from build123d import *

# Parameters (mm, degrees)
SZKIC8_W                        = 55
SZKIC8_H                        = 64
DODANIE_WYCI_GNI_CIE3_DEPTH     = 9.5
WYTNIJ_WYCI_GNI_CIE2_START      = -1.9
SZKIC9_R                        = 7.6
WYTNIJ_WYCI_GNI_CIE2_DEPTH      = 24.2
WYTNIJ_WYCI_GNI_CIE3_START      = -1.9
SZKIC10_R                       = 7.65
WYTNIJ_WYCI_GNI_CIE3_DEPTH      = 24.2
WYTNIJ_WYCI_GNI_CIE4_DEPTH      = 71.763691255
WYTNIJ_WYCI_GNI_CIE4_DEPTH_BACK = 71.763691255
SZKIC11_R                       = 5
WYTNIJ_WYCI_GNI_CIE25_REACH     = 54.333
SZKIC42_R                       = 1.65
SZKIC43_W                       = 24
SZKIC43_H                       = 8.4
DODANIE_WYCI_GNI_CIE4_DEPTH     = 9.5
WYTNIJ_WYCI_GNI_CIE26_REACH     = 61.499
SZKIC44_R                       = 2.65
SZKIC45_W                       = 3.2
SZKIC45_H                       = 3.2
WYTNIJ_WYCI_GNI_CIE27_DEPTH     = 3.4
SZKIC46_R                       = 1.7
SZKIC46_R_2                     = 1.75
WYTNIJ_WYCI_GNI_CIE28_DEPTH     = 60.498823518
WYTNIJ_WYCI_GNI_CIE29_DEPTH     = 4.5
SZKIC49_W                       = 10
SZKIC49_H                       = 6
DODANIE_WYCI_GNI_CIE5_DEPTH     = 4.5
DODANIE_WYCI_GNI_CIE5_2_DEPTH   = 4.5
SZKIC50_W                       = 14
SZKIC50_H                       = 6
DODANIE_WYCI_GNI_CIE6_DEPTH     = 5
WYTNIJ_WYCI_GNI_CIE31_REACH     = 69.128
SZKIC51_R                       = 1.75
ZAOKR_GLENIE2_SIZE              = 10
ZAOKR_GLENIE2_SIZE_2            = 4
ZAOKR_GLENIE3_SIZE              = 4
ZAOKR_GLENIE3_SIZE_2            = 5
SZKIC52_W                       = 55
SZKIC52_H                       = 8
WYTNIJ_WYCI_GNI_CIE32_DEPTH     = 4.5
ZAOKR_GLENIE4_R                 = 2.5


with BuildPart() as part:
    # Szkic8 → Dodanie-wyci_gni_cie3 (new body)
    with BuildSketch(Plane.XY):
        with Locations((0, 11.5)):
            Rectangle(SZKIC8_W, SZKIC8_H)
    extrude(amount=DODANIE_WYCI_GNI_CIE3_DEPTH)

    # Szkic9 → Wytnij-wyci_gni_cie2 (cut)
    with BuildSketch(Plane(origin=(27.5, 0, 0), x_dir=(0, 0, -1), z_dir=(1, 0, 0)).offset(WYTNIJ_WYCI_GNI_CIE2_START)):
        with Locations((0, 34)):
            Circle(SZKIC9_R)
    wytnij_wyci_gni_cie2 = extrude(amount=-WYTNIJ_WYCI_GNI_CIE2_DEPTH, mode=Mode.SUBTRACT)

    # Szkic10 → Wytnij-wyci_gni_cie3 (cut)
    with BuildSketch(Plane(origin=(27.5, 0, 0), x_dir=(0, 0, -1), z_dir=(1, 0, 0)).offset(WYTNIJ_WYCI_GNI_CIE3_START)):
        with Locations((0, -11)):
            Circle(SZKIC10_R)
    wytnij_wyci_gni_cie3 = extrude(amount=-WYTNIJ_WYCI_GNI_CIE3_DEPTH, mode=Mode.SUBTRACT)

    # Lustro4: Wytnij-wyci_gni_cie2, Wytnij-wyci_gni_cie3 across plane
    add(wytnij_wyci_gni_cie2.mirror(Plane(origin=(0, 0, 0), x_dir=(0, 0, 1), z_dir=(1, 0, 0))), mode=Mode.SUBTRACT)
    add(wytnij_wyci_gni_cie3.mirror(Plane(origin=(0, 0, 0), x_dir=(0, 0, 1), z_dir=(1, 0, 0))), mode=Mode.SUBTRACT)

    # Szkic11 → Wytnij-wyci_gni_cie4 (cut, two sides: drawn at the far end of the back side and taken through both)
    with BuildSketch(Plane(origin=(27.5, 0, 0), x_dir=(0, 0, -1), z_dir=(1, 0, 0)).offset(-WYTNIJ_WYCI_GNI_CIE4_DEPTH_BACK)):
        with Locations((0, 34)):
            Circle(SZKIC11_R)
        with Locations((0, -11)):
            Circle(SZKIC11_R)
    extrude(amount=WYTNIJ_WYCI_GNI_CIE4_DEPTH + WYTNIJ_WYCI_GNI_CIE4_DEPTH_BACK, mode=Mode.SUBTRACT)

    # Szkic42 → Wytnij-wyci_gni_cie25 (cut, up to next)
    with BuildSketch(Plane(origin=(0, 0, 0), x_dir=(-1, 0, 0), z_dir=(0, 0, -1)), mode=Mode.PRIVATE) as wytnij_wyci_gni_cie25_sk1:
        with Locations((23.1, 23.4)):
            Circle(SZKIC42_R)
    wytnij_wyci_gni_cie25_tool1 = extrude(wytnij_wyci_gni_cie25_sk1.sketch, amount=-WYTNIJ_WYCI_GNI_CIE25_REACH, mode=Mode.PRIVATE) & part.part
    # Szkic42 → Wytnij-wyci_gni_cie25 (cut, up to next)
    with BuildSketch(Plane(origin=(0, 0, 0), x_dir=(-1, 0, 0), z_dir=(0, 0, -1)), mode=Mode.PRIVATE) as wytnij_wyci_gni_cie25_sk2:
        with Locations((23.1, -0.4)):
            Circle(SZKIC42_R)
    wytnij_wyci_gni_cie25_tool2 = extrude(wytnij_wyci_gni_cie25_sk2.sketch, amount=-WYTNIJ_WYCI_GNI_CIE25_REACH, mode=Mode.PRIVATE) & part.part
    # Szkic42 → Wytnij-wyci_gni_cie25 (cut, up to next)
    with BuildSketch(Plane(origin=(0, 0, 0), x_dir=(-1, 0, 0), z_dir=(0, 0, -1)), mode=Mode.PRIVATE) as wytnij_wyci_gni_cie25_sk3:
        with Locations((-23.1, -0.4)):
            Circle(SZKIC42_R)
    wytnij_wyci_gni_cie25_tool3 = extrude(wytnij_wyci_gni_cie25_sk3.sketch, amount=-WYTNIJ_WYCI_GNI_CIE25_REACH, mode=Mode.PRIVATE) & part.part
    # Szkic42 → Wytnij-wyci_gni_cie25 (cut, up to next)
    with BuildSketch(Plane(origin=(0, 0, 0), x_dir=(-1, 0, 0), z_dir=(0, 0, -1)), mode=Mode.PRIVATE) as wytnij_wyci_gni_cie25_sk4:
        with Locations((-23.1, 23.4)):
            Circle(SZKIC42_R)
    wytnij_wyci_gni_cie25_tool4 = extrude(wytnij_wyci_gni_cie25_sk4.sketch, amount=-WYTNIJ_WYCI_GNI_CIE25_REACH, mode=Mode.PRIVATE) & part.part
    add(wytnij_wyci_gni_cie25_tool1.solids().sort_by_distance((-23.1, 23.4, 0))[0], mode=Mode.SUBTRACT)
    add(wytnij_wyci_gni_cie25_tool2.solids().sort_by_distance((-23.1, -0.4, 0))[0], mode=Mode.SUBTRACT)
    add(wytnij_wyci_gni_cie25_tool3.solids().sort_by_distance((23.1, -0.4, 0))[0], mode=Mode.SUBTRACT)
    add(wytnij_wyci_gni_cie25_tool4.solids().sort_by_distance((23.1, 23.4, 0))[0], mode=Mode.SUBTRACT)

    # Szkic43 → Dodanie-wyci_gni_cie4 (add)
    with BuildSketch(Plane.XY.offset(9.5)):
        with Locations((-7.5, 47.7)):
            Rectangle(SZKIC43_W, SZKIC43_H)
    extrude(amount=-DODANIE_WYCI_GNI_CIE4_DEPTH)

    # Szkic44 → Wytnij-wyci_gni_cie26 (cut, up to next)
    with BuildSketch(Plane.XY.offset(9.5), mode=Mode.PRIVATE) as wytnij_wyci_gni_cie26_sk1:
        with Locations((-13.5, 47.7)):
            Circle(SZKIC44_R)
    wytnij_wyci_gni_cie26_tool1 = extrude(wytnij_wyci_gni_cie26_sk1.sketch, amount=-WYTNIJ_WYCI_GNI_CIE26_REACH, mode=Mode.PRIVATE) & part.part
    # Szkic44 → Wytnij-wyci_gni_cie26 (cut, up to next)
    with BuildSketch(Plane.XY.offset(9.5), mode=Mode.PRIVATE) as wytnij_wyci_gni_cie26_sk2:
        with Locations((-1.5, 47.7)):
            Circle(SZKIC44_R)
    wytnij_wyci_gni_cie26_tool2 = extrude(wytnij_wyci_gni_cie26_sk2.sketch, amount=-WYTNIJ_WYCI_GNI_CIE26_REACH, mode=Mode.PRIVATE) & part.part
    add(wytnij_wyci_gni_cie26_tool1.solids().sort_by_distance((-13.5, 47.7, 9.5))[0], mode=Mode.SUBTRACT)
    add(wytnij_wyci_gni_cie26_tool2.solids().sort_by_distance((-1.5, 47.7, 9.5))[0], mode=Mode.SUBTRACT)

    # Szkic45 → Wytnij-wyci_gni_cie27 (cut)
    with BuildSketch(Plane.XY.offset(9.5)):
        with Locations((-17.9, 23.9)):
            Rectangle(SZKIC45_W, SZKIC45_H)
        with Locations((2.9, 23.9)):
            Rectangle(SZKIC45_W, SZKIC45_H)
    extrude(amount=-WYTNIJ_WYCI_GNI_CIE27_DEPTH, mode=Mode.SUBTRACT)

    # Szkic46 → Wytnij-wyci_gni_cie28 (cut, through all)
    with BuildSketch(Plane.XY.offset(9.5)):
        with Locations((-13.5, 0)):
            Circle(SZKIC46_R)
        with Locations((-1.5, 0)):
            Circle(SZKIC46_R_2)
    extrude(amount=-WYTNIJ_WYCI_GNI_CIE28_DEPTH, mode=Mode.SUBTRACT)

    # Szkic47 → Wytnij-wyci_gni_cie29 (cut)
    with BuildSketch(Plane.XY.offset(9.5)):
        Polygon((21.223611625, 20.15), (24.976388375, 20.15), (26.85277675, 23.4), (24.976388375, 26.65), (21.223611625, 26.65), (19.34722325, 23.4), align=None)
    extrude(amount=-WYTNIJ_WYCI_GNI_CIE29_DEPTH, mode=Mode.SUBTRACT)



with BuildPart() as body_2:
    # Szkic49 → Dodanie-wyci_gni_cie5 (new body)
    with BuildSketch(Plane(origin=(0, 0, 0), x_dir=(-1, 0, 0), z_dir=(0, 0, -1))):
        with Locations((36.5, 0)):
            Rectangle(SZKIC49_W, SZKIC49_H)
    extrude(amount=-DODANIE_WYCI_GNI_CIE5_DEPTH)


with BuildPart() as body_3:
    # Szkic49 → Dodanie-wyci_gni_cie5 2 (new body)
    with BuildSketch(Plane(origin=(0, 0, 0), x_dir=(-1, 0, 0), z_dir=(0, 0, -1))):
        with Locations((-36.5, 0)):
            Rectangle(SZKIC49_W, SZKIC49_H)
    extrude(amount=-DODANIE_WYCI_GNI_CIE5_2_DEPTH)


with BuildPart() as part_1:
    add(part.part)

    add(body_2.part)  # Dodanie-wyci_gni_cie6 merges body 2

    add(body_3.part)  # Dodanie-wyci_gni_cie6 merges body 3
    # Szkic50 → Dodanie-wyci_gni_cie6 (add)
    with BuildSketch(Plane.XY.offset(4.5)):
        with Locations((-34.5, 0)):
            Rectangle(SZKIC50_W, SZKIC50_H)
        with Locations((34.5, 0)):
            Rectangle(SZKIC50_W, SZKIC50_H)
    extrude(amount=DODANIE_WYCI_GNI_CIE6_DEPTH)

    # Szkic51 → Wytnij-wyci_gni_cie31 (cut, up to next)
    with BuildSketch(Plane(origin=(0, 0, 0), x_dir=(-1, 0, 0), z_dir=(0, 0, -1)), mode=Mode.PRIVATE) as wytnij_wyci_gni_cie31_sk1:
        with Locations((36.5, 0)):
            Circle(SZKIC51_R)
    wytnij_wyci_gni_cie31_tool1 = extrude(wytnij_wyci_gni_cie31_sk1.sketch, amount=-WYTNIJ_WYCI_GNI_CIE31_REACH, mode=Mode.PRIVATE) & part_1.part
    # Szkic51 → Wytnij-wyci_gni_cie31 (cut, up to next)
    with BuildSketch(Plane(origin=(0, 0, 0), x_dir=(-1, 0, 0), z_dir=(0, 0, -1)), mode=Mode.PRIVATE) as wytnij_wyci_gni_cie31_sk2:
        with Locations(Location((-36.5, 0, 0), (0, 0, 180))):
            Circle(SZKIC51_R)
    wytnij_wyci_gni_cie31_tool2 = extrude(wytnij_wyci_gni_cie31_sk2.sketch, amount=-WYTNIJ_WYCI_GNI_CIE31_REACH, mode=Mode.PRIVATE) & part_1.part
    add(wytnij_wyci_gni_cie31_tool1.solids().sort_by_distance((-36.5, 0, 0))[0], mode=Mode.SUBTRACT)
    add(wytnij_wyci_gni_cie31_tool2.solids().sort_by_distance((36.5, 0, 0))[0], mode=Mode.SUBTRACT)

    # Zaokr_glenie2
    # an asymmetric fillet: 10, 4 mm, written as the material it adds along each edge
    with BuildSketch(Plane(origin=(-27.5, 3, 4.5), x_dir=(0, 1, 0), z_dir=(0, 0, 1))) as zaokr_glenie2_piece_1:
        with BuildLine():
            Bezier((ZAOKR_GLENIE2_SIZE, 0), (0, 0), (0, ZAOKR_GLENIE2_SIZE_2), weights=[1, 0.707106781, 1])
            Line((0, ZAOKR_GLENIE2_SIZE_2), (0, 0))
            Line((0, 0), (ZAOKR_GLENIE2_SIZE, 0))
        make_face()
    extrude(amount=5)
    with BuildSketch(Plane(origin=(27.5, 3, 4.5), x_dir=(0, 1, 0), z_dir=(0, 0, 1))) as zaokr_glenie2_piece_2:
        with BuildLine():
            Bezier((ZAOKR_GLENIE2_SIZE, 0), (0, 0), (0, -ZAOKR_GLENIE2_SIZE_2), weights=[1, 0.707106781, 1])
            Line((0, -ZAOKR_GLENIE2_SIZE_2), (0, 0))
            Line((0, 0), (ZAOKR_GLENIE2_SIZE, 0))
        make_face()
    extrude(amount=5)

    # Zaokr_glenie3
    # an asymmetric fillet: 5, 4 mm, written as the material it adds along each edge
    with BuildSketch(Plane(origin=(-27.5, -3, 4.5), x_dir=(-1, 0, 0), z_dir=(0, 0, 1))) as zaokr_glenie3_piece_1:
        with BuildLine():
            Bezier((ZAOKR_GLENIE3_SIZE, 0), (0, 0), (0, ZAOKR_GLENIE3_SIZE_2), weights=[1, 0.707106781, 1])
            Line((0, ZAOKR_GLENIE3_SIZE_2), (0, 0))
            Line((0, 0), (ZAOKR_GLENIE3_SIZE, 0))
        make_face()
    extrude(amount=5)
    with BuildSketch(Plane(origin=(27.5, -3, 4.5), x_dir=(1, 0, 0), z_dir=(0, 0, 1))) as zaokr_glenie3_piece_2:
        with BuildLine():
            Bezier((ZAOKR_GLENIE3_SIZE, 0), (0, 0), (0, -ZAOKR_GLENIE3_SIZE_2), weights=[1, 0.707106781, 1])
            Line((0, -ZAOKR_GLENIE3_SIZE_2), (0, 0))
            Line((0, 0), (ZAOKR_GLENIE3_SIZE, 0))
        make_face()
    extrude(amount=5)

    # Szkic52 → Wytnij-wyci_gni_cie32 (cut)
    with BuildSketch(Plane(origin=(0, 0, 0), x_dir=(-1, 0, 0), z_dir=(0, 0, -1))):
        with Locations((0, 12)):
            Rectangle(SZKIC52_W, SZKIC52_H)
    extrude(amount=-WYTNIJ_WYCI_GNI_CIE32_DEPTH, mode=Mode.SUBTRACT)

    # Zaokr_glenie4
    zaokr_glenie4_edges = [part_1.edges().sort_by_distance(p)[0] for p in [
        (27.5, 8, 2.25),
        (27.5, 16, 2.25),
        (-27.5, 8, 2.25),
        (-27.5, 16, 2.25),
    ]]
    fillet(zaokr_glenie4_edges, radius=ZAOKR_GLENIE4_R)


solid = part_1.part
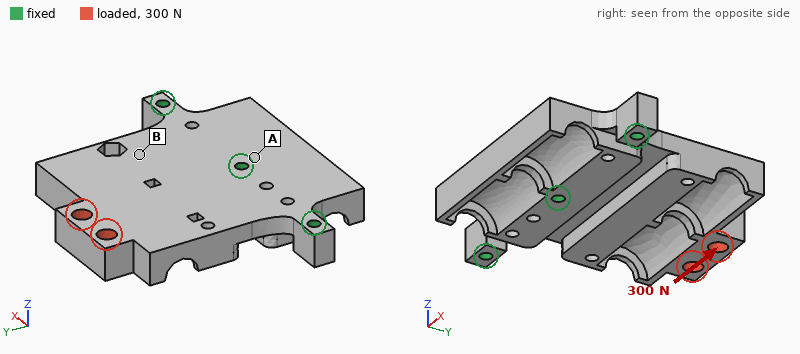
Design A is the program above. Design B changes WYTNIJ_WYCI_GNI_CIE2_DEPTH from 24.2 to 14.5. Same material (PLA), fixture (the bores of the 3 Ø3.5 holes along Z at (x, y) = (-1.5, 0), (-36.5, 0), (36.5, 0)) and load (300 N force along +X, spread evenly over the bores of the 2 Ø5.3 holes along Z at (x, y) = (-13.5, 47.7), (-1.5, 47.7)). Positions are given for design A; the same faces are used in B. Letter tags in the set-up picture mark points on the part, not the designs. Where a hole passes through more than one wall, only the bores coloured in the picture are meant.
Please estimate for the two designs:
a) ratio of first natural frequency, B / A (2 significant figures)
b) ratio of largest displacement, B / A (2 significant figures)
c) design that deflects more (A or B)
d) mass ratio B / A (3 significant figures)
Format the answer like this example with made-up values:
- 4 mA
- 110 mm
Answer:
- 1.0
- 0.82
- A
- 1.04
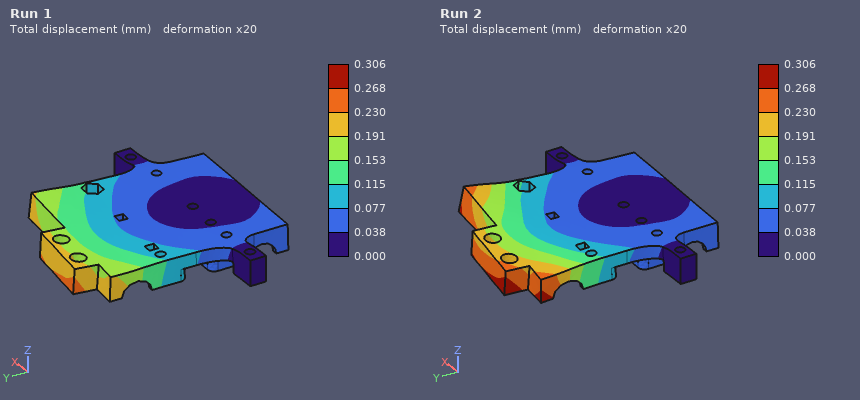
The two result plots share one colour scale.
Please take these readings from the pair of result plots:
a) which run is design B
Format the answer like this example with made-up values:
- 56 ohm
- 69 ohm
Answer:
- Run 1
